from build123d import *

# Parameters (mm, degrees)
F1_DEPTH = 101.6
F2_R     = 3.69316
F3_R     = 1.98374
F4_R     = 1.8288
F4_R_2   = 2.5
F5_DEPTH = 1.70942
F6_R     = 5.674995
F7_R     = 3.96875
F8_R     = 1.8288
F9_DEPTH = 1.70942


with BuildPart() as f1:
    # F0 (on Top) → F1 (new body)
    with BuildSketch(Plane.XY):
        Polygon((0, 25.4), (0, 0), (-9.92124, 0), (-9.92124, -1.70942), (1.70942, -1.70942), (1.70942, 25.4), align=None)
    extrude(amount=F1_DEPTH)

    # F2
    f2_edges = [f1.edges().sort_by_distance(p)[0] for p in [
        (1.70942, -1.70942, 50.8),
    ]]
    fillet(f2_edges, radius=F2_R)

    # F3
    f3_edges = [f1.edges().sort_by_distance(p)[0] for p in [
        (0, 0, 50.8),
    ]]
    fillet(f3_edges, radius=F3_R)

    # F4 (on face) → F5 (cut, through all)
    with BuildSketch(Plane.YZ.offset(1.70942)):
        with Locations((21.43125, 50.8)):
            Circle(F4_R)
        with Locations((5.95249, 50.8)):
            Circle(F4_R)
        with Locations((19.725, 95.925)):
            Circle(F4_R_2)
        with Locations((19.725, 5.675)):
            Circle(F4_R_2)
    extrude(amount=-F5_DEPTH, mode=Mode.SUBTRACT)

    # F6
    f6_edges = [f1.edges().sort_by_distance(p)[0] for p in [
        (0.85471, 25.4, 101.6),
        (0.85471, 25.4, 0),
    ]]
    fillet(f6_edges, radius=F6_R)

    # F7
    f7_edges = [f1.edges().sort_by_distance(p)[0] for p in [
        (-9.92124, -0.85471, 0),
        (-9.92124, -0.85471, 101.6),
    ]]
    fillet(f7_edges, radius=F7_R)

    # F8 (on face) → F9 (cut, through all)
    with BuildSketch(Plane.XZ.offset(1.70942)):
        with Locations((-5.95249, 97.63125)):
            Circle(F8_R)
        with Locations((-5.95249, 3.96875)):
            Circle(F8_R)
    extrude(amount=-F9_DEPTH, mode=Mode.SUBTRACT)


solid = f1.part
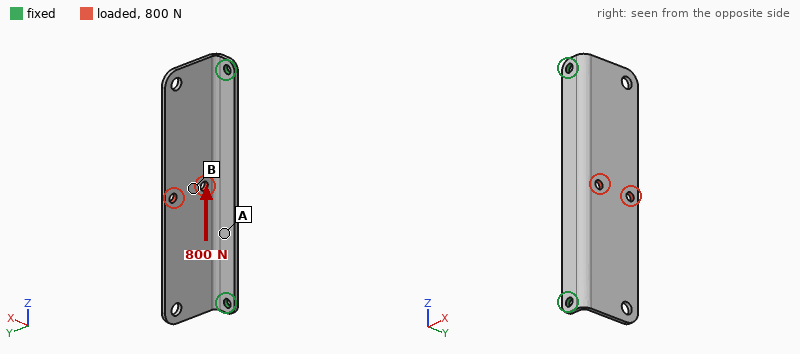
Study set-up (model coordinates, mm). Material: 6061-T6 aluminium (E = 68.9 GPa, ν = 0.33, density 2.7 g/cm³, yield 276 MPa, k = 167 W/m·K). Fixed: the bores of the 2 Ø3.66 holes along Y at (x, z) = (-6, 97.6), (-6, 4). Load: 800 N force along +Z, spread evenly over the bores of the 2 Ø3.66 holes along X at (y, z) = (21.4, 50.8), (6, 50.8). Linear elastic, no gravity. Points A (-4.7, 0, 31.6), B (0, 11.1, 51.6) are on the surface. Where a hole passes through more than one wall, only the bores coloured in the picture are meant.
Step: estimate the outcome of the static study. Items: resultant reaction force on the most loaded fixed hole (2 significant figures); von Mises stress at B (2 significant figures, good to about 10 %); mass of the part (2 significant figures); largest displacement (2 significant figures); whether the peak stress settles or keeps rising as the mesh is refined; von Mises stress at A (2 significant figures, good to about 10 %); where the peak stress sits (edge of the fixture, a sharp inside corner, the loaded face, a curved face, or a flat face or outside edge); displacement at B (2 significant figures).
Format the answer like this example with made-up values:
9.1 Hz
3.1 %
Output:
420 N
6.8 MPa
16 g
84 µm
keeps rising
12 MPa
edge of the fixture
15 µm
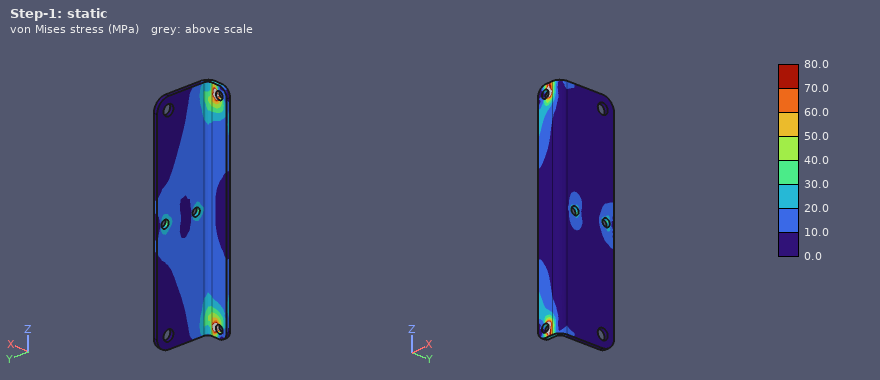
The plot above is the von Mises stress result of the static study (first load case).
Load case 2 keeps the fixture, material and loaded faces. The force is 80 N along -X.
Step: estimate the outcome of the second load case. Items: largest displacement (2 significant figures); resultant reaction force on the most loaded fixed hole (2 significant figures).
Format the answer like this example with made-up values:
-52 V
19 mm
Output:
0.54 mm
59 N
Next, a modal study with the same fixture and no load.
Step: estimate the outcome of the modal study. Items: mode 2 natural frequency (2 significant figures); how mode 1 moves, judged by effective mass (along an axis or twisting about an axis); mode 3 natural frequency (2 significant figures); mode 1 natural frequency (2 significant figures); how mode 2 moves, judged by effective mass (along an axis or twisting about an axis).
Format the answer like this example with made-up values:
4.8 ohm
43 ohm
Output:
1800 Hz
along X
2700 Hz
910 Hz
twisting about Y
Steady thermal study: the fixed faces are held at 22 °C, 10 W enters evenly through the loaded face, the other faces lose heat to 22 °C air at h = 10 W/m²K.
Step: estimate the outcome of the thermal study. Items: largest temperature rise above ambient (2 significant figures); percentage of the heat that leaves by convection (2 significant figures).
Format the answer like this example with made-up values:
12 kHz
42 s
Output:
34 K
13 %
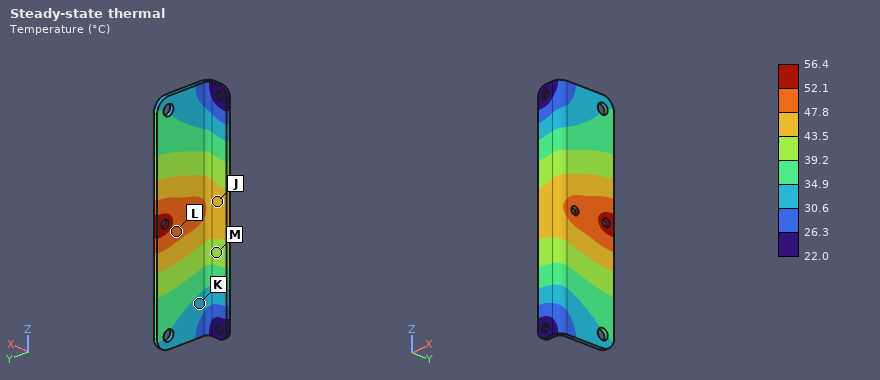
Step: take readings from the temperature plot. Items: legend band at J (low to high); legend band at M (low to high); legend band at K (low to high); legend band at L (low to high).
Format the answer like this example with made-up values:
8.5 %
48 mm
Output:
43.5 to 47.8 °C
39.2 to 43.5 °C
30.6 to 34.9 °C
47.8 to 52.1 °C
